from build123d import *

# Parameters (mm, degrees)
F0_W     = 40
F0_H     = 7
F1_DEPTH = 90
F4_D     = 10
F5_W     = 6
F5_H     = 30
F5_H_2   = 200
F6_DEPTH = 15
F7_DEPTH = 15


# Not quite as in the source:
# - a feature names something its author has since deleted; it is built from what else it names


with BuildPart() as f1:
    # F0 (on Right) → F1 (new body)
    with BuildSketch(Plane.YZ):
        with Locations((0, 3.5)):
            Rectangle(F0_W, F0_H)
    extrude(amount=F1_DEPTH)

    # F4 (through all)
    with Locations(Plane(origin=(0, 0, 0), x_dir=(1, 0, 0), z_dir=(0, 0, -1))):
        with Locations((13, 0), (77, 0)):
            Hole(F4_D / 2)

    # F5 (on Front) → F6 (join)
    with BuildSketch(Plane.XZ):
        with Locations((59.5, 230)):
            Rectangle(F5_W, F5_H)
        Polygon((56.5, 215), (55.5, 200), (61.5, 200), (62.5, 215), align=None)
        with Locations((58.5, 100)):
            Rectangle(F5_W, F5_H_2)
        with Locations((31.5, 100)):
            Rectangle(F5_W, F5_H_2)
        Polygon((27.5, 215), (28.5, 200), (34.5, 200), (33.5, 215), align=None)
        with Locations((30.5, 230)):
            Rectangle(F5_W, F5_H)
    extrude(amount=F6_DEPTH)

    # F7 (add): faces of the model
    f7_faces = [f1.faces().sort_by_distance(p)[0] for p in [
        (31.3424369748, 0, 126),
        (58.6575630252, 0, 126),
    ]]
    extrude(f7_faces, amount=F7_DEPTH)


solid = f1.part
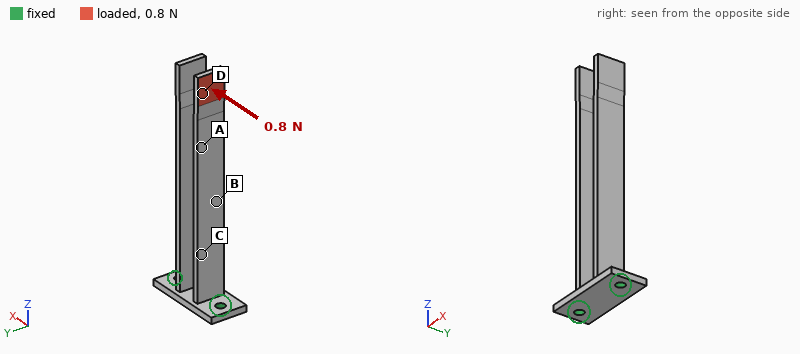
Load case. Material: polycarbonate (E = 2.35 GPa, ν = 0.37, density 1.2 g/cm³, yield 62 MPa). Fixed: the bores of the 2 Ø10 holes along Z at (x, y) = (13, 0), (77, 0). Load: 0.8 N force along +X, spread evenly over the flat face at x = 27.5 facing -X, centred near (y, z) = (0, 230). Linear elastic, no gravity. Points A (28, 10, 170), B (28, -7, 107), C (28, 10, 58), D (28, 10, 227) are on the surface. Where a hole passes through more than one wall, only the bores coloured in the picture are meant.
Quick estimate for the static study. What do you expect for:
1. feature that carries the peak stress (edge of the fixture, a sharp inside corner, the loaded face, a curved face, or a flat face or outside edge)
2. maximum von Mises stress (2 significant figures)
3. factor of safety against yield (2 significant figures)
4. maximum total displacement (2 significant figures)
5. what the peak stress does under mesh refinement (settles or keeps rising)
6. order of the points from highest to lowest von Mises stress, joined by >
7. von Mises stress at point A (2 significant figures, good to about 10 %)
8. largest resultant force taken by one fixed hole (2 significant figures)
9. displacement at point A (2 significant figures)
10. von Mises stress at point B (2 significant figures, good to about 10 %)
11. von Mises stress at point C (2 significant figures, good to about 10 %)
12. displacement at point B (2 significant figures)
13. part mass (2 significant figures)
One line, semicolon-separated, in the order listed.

a flat face or outside edge; 0.97 MPa; 64; 2.7 mm; settles; C > B > A > D; 0.27 MPa; 3.6 N; 1.5 mm; 0.55 MPa; 0.77 MPa; 0.64 mm; 130 g
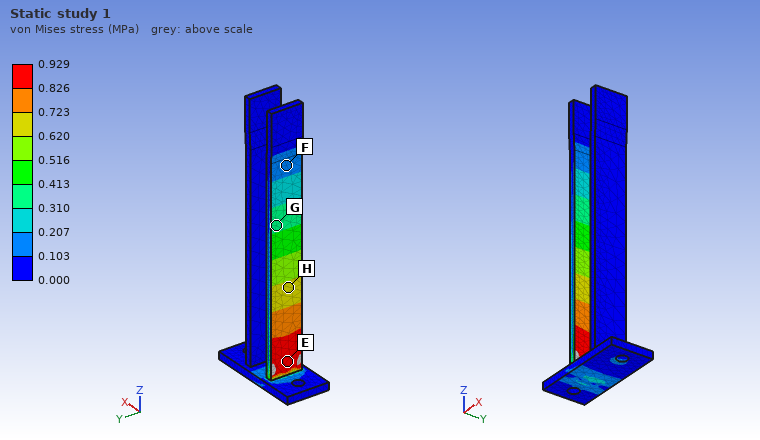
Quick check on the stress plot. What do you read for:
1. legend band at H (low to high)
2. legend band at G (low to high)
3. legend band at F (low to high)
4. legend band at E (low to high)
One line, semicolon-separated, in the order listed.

0.620 to 0.723 MPa; 0.310 to 0.413 MPa; 0.103 to 0.207 MPa; 0.826 to 0.929 MPa
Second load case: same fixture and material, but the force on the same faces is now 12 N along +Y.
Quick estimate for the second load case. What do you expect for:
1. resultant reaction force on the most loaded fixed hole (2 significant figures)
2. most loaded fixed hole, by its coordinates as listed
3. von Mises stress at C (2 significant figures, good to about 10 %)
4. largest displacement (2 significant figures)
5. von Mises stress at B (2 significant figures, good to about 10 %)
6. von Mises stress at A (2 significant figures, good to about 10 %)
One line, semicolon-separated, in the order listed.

9.8 N; (13, 0); 1.6 MPa; 2.9 mm; 0.84 MPa; 0.65 MPa
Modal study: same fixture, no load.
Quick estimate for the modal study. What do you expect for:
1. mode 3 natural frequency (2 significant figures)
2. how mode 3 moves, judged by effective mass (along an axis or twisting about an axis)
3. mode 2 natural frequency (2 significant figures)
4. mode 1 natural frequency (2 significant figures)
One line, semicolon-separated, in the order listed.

71 Hz; along Y; 24 Hz; 23 Hz
